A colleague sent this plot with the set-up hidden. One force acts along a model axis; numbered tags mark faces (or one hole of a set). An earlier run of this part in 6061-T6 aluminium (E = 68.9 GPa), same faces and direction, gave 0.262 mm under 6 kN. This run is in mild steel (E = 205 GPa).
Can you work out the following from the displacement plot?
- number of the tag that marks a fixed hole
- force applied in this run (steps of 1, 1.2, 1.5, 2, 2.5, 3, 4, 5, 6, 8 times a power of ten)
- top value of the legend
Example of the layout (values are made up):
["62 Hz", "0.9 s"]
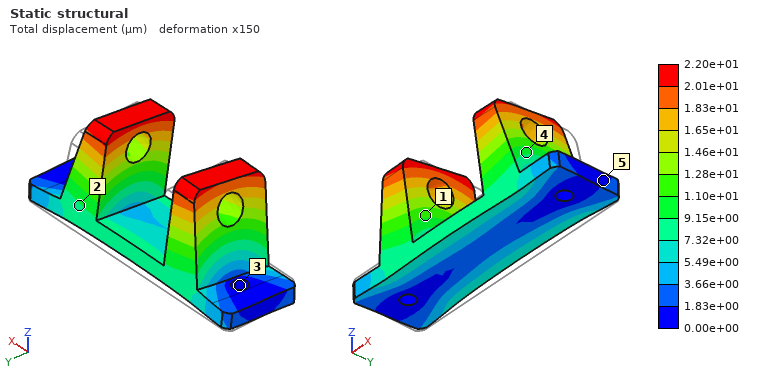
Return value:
["3", "1.5 kN", "2.20e+01 µm"]
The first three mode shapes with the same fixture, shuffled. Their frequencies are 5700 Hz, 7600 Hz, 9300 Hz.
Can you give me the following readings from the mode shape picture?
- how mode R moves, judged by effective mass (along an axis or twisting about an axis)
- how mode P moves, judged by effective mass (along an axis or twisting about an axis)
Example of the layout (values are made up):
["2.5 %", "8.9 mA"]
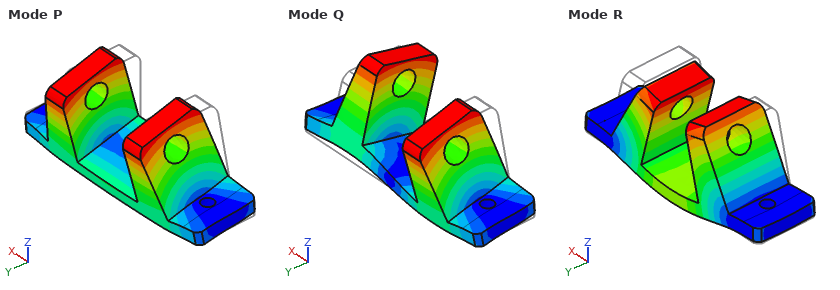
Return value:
["along Z", "along Y"]
